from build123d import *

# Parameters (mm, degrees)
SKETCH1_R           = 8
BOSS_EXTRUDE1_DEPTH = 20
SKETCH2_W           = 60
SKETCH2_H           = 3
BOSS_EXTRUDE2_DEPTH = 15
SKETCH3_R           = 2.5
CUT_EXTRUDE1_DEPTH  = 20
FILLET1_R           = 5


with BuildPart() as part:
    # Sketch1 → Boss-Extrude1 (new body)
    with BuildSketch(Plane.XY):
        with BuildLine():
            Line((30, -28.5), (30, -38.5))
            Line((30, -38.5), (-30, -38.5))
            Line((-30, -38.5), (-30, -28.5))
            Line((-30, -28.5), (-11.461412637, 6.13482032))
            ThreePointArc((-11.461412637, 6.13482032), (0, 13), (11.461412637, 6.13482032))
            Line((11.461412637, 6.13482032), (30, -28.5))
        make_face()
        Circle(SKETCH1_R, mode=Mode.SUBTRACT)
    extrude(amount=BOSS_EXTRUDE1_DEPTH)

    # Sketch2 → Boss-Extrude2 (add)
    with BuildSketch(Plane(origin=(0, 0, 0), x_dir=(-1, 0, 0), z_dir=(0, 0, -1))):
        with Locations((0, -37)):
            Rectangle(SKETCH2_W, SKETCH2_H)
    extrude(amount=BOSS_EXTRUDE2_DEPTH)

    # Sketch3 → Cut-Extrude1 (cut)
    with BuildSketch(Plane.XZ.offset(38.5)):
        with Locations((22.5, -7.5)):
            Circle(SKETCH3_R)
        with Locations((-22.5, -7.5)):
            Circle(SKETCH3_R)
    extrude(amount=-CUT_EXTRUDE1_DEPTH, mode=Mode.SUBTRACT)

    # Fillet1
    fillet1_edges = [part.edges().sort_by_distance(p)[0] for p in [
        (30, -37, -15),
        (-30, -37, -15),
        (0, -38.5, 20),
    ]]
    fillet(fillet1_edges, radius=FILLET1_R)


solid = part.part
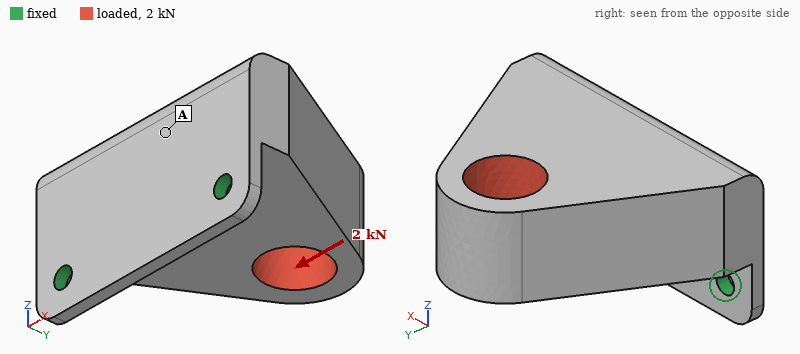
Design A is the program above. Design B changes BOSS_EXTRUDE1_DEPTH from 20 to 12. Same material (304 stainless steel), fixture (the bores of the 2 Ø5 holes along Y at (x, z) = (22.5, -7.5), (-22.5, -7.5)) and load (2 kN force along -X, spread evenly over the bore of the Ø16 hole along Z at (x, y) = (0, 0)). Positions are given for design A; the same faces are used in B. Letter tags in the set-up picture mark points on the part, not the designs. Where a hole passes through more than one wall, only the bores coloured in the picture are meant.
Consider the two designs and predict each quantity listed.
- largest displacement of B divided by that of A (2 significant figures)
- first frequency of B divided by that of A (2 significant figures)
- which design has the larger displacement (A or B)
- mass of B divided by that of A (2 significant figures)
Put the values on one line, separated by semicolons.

1.1; 1.4; B; 0.62
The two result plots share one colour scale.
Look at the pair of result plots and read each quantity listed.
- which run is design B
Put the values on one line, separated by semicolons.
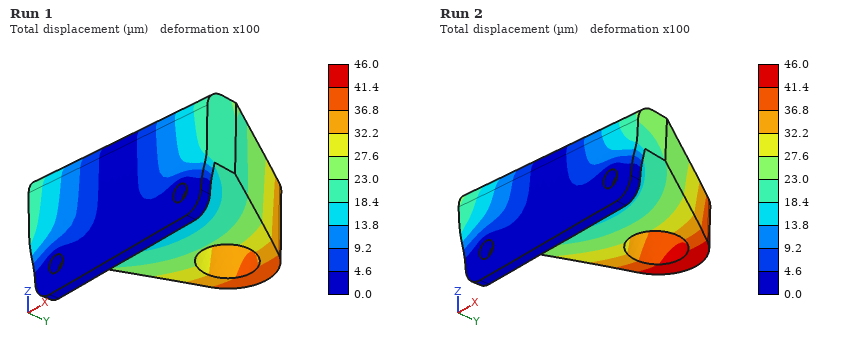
Run 2
